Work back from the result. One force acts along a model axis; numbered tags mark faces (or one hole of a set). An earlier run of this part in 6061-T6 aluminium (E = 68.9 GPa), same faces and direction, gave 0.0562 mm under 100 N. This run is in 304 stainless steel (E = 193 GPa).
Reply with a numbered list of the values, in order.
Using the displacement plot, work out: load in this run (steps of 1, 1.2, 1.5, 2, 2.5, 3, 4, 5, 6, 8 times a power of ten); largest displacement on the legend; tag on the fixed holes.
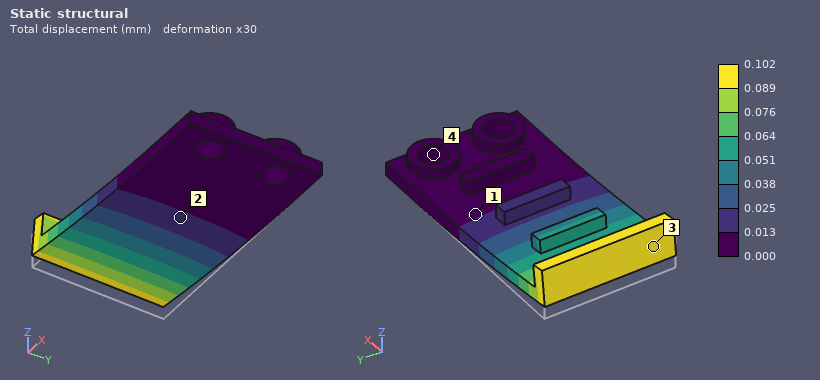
1. 500 N
2. 0.102 mm
3. 4
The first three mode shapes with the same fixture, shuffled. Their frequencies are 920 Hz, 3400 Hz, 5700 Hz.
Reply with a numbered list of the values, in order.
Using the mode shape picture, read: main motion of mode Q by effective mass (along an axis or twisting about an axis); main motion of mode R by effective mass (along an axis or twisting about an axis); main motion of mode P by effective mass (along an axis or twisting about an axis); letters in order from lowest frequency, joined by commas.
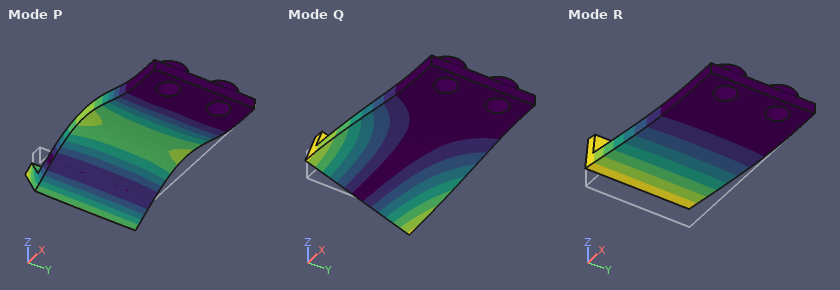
1. twisting about X
2. along Z
3. along Z
4. R, Q, P
